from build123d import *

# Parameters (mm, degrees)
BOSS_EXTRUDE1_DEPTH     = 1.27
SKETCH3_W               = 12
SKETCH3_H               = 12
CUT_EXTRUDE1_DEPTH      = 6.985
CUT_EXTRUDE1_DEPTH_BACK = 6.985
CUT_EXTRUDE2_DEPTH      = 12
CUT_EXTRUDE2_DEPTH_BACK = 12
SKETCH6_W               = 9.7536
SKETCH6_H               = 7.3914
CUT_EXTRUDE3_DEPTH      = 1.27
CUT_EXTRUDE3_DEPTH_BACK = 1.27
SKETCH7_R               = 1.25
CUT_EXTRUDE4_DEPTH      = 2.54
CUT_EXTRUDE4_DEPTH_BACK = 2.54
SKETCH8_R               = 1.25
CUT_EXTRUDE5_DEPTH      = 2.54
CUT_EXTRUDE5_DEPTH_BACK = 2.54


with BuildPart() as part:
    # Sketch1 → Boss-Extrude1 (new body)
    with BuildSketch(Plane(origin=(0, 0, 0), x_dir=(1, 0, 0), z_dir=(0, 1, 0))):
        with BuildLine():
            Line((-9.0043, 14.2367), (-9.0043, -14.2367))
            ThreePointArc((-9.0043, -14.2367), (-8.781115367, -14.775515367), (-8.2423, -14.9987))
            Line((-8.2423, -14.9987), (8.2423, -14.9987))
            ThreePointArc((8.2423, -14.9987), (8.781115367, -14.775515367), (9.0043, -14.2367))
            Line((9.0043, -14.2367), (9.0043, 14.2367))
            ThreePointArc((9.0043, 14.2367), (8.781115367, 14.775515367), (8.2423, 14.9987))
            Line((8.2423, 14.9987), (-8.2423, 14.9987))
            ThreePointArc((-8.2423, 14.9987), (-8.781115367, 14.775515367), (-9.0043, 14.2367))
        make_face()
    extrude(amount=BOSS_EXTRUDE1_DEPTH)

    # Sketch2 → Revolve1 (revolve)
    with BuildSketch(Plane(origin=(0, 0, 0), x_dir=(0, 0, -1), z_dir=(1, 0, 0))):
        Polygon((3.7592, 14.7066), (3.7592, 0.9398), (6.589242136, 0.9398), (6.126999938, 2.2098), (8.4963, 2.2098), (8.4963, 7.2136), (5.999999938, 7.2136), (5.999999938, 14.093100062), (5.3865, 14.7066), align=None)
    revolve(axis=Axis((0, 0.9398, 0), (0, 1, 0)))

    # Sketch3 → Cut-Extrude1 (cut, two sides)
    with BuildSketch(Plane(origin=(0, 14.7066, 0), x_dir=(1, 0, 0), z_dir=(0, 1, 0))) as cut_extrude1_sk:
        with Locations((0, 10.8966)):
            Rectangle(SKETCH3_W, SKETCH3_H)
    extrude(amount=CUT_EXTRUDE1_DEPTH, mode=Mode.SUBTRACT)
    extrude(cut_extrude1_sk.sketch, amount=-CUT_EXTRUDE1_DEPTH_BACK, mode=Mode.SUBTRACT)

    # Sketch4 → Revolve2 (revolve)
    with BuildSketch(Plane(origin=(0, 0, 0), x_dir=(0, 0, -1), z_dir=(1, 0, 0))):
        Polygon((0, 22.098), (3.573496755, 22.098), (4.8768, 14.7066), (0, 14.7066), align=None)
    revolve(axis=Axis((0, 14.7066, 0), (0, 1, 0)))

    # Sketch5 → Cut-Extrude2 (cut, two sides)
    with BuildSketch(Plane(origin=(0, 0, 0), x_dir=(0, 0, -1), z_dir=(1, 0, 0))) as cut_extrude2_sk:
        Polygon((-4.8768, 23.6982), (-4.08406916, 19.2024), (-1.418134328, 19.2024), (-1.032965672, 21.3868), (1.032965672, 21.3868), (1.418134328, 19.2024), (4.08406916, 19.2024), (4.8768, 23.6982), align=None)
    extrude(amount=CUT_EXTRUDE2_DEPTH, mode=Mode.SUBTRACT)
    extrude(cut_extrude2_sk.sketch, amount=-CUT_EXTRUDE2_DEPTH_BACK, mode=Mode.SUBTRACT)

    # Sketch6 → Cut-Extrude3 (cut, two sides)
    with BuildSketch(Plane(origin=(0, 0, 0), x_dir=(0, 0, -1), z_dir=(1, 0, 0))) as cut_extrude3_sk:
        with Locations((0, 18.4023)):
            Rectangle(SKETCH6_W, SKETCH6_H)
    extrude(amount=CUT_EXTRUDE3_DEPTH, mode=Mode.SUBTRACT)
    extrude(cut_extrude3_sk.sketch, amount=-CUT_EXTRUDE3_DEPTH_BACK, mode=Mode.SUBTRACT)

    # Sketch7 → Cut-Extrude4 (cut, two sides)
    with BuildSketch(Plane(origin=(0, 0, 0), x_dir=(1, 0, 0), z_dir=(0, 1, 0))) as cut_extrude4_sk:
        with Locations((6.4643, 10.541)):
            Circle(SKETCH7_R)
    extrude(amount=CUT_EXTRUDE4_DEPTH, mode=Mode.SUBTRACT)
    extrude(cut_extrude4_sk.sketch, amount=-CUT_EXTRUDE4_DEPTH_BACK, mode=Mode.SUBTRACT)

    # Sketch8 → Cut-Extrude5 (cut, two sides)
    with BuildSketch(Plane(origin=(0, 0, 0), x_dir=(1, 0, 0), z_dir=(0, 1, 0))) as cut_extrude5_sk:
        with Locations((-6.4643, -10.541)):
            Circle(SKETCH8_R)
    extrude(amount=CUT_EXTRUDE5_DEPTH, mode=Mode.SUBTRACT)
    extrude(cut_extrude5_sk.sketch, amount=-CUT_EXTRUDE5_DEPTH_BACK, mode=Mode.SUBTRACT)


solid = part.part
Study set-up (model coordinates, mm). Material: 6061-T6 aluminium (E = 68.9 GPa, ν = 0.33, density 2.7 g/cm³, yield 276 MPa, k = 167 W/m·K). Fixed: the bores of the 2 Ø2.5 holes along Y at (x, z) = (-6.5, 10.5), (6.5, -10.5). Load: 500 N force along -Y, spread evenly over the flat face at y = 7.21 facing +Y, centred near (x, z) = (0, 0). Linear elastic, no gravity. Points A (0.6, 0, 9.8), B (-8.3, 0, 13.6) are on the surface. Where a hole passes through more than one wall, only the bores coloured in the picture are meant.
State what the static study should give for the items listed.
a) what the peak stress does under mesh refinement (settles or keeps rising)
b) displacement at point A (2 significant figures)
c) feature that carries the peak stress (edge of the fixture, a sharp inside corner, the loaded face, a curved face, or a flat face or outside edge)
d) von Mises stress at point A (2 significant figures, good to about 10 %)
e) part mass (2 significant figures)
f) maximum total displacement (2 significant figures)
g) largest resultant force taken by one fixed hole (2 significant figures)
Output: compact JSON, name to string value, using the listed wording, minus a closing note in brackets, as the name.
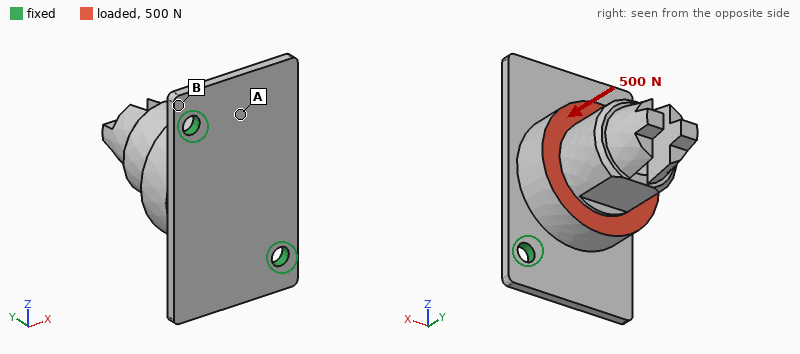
{"what the peak stress does under mesh refinement": "keeps rising", "displacement at point A": "36 µm", "feature that carries the peak stress": "edge of the fixture", "von Mises stress at point A": "49 MPa", "part mass": "6.3 g", "maximum total displacement": "58 µm", "largest resultant force taken by one fixed hole": "270 N"}
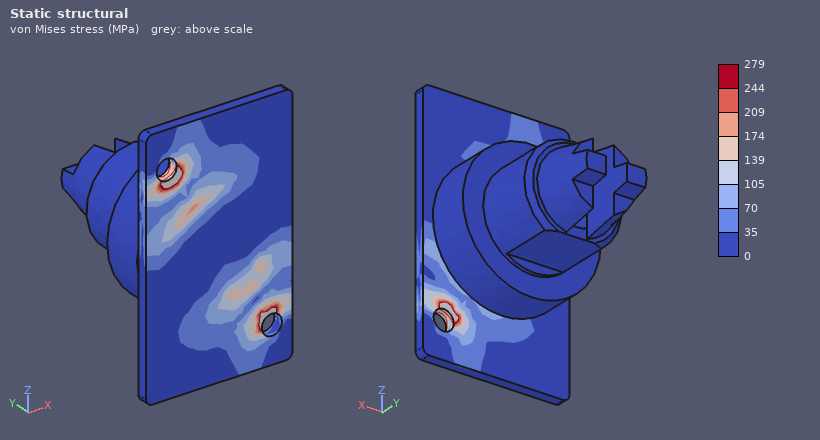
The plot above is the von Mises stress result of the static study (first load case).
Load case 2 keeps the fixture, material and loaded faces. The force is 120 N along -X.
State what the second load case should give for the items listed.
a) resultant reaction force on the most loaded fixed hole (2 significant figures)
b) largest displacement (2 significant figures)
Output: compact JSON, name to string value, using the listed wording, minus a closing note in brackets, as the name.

{"resultant reaction force on the most loaded fixed hole": "64 N", "largest displacement": "0.17 mm"}
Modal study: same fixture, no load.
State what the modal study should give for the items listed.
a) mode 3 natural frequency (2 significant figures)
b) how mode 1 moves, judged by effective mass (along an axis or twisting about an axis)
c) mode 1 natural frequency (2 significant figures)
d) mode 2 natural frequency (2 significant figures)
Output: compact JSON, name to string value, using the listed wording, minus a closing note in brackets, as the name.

{"mode 3 natural frequency": "6700 Hz", "how mode 1 moves, judged by effective mass": "along X", "mode 1 natural frequency": "2100 Hz", "mode 2 natural frequency": "6400 Hz"}
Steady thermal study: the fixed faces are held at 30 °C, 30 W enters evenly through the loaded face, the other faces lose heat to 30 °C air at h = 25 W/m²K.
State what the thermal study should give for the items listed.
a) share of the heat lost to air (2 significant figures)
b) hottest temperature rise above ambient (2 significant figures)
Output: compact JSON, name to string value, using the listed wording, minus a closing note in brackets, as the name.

{"share of the heat lost to air": "8.0 %", "hottest temperature rise above ambient": "53 K"}
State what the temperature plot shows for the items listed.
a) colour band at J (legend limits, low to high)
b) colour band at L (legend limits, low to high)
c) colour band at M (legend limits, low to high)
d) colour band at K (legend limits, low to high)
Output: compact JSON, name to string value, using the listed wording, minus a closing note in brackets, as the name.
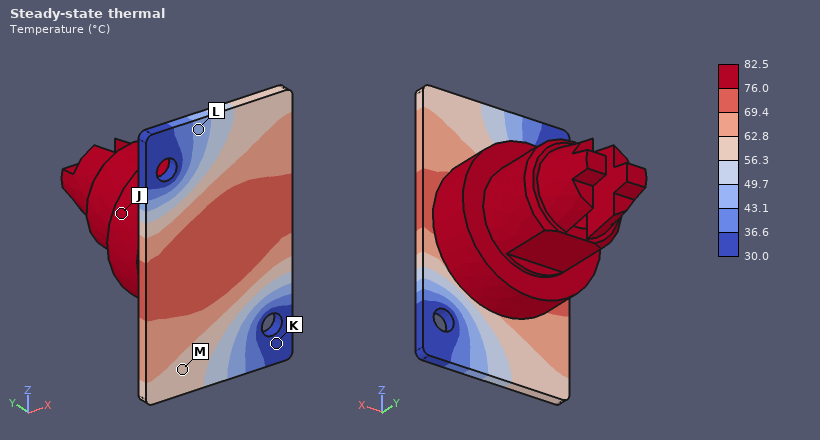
{"colour band at J": "76.0 to 82.5 °C", "colour band at L": "43.1 to 49.7 °C", "colour band at M": "56.3 to 62.8 °C", "colour band at K": "30.0 to 36.6 °C"}
